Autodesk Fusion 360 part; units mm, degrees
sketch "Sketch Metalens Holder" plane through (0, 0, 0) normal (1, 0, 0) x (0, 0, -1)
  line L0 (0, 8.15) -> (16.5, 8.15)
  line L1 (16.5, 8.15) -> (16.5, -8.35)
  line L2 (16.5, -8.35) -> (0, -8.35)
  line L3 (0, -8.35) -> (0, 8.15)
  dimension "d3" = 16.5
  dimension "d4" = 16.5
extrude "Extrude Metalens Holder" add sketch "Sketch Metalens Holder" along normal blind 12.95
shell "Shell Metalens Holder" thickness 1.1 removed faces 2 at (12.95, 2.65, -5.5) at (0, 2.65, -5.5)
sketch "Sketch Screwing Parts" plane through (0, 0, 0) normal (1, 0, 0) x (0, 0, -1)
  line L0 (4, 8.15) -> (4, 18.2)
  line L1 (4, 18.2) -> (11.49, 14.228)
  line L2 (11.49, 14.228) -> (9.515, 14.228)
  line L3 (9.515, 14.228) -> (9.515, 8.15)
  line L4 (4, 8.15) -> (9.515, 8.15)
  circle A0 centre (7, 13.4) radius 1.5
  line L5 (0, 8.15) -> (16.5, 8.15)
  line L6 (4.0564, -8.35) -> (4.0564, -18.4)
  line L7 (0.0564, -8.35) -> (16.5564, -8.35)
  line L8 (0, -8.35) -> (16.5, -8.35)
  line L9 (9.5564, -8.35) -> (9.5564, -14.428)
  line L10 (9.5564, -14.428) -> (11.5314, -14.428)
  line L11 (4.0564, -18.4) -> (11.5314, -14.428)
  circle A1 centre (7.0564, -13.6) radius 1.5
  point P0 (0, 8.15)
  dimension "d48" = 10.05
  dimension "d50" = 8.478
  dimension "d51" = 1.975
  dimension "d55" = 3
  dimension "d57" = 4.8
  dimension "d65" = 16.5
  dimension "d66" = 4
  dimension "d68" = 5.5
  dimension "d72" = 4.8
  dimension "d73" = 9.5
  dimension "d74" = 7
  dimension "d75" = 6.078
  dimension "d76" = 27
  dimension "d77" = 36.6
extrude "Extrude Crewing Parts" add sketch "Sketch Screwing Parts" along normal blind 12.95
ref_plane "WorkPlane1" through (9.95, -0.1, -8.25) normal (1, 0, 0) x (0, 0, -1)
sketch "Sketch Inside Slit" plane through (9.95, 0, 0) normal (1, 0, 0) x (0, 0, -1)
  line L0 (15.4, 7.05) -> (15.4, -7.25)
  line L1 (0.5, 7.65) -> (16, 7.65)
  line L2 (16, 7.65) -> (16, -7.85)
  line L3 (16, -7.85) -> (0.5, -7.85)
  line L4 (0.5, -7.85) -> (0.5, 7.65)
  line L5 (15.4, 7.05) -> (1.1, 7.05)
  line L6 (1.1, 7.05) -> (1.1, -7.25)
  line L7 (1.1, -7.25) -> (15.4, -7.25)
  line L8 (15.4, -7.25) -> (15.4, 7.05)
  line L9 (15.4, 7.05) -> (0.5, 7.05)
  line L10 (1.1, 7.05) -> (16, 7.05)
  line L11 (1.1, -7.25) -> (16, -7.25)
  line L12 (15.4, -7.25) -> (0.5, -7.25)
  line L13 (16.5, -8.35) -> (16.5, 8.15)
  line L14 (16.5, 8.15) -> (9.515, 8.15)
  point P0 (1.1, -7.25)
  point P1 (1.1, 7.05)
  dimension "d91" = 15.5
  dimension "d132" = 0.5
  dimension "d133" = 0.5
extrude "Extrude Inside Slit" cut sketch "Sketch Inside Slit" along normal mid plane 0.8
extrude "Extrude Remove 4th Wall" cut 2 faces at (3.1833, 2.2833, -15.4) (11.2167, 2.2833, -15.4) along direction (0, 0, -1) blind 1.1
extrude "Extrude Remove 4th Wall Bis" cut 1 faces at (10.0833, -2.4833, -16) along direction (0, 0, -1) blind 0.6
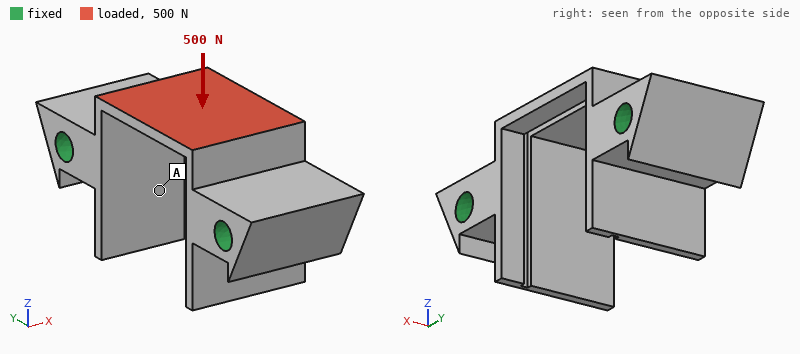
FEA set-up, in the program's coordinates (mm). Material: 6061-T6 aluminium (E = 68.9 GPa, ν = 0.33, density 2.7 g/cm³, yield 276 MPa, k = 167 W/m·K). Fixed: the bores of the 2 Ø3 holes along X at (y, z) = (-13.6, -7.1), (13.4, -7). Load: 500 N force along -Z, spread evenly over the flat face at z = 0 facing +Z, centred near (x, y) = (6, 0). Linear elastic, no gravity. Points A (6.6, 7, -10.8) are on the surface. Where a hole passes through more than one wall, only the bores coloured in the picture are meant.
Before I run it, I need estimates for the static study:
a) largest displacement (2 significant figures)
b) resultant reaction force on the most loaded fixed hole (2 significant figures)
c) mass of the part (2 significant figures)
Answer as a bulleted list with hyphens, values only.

- 65 µm
- 320 N
- 4.6 g
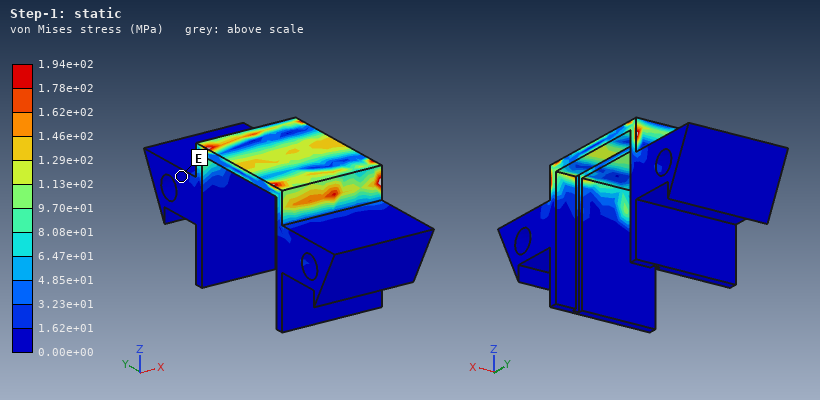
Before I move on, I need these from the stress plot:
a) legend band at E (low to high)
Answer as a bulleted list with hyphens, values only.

- 0.00e+00 to 1.62e+01 MPa
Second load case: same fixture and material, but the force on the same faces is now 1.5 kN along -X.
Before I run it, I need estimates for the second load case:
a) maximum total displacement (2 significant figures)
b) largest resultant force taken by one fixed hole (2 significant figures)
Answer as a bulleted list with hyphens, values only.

- 49 µm
- 750 N
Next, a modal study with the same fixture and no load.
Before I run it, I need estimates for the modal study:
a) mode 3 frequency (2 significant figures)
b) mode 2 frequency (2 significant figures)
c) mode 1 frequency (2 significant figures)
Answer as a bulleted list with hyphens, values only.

- 22 kHz
- 16 kHz
- 16 kHz
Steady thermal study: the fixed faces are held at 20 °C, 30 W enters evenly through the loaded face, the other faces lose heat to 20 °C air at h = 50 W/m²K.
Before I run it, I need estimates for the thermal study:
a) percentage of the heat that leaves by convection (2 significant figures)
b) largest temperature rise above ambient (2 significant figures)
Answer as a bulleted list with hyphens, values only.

- 3.2 %
- 54 K
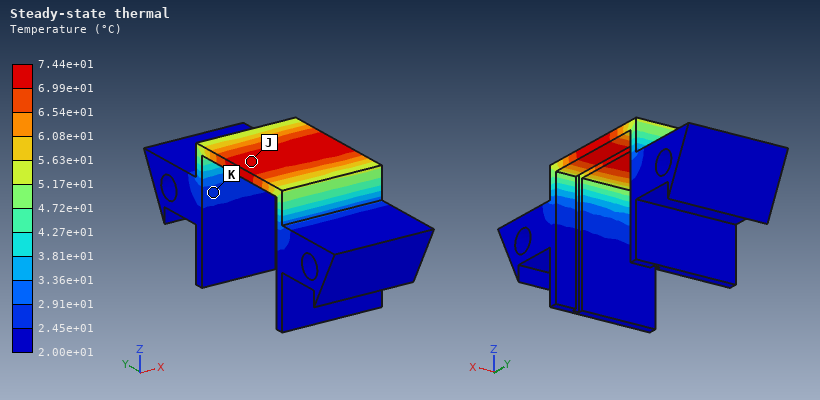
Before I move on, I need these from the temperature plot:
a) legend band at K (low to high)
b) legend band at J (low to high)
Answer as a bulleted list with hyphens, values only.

- 2.45e+01 to 2.91e+01 °C
- 6.99e+01 to 7.44e+01 °C
